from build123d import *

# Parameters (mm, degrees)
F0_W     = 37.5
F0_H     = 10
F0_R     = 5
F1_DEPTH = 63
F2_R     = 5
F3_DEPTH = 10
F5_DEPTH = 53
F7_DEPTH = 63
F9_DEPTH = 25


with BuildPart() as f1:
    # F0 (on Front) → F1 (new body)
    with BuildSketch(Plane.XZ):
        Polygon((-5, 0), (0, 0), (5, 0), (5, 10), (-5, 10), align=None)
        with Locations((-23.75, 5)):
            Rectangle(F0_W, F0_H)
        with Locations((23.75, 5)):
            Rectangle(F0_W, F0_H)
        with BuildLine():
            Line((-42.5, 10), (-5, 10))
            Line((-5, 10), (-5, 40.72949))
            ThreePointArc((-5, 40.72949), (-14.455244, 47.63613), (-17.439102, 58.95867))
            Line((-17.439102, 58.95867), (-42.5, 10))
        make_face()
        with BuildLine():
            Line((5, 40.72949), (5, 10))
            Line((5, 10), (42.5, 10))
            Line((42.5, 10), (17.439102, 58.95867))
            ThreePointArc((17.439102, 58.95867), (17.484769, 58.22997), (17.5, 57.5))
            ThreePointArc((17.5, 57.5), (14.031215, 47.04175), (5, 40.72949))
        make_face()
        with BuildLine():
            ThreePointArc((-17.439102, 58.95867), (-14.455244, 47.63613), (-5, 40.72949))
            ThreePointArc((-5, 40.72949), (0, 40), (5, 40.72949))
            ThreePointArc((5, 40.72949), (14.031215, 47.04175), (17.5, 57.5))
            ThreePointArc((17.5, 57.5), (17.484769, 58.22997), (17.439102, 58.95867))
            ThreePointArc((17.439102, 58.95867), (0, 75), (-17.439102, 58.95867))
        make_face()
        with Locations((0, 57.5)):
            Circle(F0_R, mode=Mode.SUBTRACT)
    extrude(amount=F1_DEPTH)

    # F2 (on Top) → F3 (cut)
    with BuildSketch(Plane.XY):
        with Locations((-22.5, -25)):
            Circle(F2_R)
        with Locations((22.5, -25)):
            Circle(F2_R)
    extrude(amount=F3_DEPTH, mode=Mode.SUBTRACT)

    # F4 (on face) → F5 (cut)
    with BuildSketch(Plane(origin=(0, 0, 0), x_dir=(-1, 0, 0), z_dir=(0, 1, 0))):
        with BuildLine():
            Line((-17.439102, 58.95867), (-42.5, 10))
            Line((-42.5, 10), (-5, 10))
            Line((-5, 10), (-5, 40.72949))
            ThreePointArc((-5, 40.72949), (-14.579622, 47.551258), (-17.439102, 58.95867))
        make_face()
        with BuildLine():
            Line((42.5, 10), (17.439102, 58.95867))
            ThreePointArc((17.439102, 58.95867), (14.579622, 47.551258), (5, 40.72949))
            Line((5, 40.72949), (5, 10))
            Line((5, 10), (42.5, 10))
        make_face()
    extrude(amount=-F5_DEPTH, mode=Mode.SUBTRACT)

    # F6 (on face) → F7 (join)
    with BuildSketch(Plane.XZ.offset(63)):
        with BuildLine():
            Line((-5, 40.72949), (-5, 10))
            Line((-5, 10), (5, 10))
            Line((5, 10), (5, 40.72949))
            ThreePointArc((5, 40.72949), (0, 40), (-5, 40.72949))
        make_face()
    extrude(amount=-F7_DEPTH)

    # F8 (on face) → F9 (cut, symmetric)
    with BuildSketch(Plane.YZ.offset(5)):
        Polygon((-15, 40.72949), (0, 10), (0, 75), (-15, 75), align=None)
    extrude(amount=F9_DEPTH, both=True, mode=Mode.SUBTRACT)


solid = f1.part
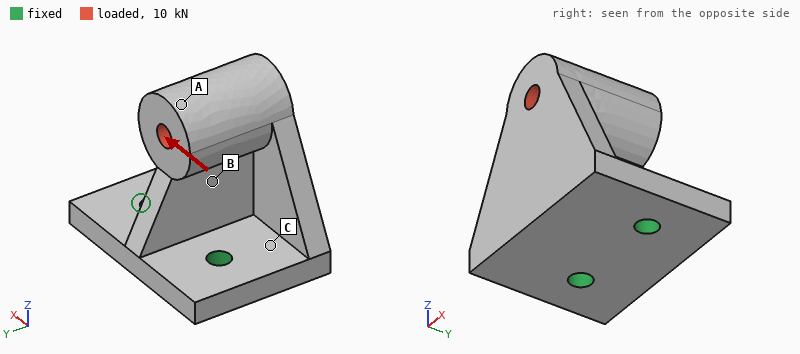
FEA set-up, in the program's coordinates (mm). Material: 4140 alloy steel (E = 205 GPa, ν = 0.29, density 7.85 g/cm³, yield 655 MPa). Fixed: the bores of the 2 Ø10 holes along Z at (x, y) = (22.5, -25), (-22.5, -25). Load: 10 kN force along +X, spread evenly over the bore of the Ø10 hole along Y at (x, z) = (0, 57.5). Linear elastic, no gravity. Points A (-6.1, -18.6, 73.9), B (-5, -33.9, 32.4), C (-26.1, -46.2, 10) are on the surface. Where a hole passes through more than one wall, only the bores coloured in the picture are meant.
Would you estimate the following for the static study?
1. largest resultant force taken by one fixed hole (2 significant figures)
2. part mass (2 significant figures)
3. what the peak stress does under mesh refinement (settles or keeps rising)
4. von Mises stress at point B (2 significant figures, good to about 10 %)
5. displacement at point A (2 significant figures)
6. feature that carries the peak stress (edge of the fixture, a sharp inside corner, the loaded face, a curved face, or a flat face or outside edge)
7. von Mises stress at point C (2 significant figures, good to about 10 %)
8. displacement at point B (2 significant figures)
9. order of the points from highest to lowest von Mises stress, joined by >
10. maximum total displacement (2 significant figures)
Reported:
13 kN
1.0 kg
keeps rising
47 MPa
0.18 mm
edge of the fixture
84 MPa
0.062 mm
C > B > A
0.18 mm
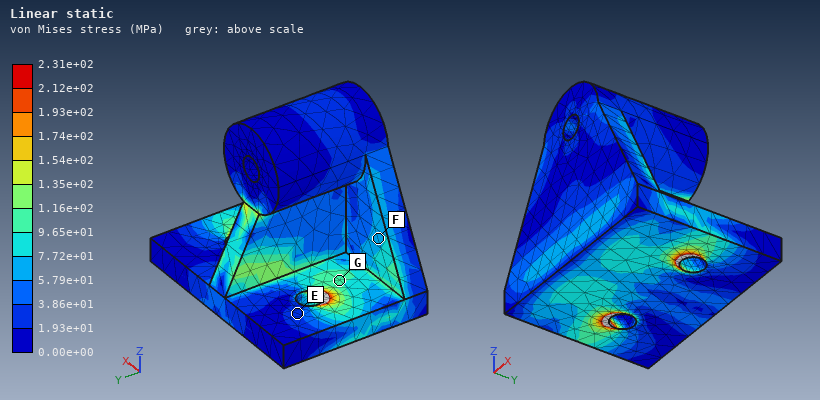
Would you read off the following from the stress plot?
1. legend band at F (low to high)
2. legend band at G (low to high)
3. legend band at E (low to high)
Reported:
5.79e+01 to 7.72e+01 MPa
9.65e+01 to 1.16e+02 MPa
1.93e+01 to 3.86e+01 MPa
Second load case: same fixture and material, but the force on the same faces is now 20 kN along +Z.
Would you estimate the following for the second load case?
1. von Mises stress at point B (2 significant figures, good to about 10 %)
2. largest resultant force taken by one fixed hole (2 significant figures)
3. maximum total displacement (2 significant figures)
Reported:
45 MPa
10 kN
99 µm
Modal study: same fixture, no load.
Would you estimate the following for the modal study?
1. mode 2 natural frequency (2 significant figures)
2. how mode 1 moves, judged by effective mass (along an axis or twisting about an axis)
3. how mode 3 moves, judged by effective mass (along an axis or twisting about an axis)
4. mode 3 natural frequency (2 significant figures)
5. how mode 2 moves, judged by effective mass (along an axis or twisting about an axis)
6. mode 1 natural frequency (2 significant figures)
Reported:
2200 Hz
along Y
twisting about Z
5500 Hz
along X
1800 Hz
